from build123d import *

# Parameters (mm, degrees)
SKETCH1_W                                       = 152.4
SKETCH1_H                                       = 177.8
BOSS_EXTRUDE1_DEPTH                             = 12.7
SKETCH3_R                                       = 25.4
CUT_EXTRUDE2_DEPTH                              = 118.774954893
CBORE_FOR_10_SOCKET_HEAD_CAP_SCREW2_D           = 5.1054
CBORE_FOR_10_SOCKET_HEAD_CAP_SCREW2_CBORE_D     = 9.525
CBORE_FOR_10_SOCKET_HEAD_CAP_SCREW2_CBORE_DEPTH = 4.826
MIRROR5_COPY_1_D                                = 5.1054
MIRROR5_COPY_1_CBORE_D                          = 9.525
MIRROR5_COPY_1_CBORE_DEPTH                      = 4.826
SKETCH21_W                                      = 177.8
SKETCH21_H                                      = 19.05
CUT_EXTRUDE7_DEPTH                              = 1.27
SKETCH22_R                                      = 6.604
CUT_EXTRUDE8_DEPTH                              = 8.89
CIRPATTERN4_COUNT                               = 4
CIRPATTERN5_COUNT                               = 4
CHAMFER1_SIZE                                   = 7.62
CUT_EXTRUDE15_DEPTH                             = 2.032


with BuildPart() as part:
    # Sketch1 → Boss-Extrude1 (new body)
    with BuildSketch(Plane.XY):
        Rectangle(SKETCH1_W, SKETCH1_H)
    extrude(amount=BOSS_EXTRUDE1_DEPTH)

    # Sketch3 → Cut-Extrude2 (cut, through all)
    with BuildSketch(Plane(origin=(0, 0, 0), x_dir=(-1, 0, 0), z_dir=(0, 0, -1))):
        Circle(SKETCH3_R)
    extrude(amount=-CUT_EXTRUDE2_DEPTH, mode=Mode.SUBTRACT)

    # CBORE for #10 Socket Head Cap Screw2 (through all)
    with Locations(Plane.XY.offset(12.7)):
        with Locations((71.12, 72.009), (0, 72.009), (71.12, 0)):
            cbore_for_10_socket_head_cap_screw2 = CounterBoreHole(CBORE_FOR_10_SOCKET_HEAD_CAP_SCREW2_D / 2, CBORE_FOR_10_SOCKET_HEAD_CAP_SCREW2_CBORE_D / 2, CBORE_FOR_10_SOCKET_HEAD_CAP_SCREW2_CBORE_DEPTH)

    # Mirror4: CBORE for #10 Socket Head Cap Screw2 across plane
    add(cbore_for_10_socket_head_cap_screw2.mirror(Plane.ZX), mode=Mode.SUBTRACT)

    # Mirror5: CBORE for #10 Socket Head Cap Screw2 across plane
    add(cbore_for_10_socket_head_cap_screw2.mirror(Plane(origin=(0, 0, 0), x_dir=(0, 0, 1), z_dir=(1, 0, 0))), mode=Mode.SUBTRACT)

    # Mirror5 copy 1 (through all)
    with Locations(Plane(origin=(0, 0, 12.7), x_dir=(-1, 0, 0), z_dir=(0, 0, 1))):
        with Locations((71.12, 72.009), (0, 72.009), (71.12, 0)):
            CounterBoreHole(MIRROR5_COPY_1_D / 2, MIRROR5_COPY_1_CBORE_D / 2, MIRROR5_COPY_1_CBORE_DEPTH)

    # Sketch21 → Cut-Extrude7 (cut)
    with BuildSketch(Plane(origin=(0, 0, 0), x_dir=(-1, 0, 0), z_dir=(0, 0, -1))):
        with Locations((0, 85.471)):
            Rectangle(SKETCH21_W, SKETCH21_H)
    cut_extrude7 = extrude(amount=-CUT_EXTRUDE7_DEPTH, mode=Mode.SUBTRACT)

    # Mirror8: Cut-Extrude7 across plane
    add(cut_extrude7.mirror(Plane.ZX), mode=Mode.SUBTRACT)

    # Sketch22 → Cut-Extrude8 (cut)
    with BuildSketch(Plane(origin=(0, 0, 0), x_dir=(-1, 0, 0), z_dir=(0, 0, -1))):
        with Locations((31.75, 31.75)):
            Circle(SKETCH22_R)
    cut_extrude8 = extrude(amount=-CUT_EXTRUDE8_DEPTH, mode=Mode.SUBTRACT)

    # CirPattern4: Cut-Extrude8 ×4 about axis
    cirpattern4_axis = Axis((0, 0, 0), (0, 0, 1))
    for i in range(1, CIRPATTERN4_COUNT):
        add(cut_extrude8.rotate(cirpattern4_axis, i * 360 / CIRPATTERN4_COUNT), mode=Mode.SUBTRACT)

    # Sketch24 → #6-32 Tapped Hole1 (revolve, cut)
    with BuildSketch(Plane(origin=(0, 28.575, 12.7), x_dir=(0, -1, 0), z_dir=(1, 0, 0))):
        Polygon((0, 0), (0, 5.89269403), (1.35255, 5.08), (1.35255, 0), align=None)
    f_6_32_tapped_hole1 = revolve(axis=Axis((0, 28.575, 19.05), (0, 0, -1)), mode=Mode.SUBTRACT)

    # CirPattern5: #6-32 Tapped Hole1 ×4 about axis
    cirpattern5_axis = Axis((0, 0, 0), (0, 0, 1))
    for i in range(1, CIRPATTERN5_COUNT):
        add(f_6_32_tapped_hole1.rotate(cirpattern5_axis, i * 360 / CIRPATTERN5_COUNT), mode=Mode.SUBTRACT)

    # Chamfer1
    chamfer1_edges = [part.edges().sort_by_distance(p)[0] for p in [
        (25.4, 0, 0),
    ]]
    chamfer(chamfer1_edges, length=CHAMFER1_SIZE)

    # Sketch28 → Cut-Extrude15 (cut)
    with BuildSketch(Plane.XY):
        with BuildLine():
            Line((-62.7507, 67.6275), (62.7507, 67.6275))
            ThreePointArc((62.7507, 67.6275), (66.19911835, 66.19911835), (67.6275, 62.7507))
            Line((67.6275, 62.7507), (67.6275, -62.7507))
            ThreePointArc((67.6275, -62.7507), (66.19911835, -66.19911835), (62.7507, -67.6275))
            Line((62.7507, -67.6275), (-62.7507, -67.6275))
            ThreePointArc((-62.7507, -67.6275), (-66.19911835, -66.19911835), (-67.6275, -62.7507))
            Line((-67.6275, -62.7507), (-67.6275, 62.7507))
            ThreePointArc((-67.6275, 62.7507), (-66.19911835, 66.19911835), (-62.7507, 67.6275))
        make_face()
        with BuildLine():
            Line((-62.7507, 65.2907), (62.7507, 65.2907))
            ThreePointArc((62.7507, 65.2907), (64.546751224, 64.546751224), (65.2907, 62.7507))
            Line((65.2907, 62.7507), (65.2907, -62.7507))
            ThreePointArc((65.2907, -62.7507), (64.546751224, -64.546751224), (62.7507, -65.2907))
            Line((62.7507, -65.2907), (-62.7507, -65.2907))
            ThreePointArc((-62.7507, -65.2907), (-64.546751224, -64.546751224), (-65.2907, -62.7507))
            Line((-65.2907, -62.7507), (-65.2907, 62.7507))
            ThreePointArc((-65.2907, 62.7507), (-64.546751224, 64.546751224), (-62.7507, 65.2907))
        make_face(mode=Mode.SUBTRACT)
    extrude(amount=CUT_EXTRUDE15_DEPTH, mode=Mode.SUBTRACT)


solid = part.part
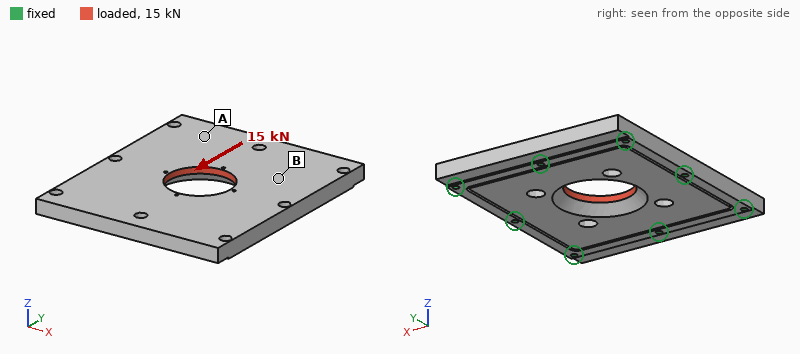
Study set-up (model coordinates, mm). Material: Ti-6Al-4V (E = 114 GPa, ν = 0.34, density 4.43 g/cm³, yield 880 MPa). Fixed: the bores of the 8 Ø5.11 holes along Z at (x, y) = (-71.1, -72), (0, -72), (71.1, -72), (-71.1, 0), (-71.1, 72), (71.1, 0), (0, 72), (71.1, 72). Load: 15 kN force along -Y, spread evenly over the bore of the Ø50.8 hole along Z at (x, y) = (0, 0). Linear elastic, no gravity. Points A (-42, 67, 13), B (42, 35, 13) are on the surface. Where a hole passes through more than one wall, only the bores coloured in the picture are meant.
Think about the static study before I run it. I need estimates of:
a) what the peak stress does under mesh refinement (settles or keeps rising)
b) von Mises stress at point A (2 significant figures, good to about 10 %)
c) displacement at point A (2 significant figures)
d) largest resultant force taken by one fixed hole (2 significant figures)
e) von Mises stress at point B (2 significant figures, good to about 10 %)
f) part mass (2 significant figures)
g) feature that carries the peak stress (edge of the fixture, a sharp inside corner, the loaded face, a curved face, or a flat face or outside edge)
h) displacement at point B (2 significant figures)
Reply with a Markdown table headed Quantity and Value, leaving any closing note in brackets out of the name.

| Quantity | Value |
|---|---|
| what the peak stress does under mesh refinement | keeps rising |
| von Mises stress at point A | 3.3 MPa |
| displacement at point A | 2.3 µm |
| largest resultant force taken by one fixed hole | 3.4 kN |
| von Mises stress at point B | 6.9 MPa |
| part mass | 1.3 kg |
| feature that carries the peak stress | edge of the fixture |
| displacement at point B | 2.7 µm |
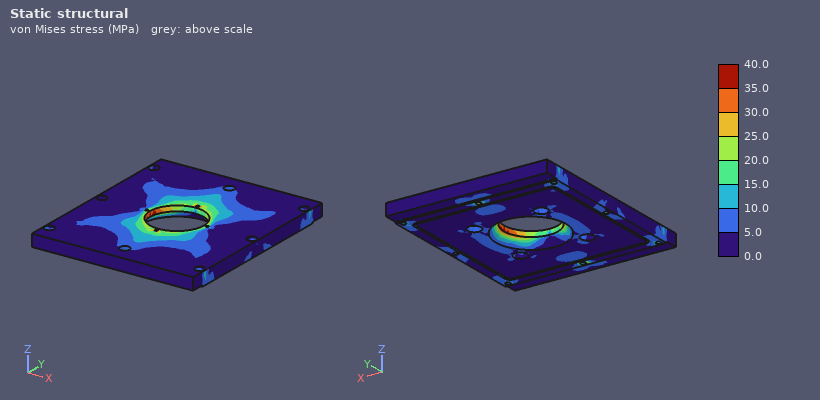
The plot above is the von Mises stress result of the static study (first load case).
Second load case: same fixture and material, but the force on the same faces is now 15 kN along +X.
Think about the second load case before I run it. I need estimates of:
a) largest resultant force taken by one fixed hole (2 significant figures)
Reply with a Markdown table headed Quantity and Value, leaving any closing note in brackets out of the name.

| Quantity | Value |
|---|---|
| largest resultant force taken by one fixed hole | 3.2 kN |
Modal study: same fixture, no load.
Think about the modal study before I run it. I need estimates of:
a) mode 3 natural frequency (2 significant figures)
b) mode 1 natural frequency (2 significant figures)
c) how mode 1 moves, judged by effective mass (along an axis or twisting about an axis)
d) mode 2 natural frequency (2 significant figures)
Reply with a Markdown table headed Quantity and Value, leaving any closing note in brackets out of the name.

| Quantity | Value |
|---|---|
| mode 3 natural frequency | 5600 Hz |
| mode 1 natural frequency | 3500 Hz |
| how mode 1 moves, judged by effective mass | along Z |
| mode 2 natural frequency | 5500 Hz |
